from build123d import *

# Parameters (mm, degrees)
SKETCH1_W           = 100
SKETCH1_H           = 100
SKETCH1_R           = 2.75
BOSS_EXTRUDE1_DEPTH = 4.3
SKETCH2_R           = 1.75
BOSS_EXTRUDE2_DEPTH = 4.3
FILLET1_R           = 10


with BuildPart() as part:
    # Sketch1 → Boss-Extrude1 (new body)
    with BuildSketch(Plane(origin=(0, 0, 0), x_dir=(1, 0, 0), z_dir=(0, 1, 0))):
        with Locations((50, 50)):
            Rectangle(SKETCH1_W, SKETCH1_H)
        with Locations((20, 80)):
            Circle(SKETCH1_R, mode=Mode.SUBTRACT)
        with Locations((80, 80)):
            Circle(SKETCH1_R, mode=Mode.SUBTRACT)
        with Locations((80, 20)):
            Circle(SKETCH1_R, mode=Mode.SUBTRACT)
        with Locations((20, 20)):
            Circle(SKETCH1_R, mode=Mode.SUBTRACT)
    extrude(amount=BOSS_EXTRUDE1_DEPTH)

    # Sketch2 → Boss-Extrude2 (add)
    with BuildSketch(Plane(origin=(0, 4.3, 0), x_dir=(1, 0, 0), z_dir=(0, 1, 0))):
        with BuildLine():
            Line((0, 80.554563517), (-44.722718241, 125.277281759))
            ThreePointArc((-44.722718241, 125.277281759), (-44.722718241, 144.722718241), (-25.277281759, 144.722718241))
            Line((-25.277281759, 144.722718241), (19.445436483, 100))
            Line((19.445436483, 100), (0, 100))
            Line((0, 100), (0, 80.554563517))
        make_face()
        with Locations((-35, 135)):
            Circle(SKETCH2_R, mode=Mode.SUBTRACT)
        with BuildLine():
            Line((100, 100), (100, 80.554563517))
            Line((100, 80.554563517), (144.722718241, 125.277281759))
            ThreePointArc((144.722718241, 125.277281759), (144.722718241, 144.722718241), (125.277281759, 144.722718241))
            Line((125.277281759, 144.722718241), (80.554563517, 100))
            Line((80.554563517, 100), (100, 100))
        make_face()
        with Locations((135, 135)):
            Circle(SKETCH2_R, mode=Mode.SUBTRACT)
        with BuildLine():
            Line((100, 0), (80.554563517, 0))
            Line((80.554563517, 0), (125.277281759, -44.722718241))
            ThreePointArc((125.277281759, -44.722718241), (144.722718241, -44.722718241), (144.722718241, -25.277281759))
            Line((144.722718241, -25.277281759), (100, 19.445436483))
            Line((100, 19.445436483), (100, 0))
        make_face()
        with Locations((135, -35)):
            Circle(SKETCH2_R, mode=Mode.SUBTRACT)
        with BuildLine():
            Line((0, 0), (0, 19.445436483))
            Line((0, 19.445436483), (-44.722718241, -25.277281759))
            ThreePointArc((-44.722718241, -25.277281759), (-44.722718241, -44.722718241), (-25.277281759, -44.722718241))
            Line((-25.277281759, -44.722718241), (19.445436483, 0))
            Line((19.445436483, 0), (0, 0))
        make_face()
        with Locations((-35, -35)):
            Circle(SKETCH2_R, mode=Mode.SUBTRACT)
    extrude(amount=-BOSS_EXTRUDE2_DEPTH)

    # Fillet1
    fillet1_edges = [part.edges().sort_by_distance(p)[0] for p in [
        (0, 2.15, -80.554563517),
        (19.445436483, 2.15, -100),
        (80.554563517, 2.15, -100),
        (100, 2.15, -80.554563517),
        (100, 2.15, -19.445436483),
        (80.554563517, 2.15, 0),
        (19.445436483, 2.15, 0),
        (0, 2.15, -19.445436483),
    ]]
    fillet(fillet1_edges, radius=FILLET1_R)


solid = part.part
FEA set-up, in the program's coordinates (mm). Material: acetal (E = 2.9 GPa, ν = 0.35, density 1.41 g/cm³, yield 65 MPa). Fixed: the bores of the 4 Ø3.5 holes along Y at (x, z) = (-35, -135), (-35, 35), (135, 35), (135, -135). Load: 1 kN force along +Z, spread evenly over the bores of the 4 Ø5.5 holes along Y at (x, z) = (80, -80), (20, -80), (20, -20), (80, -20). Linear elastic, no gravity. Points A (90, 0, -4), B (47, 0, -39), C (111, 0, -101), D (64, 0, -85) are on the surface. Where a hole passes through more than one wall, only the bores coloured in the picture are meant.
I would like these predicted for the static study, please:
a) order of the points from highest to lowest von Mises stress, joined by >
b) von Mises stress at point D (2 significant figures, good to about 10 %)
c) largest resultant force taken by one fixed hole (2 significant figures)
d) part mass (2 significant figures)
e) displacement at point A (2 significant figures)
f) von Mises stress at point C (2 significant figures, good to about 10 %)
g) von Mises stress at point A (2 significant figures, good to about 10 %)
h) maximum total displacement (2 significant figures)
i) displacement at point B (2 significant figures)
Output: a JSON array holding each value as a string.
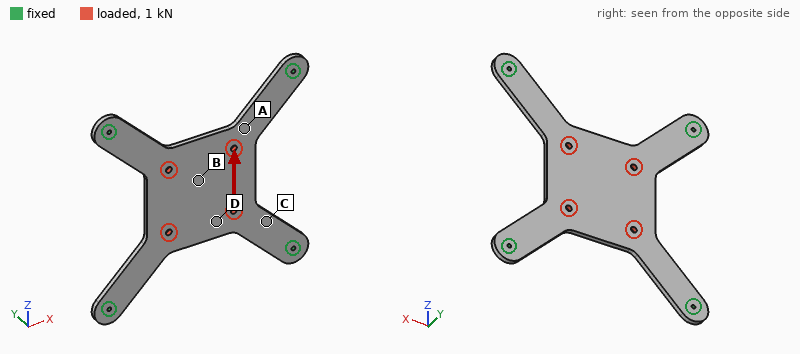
["C > A > D > B", "1.4 MPa", "340 N", "100 g", "0.12 mm", "3.3 MPa", "2.3 MPa", "0.14 mm", "0.12 mm"]
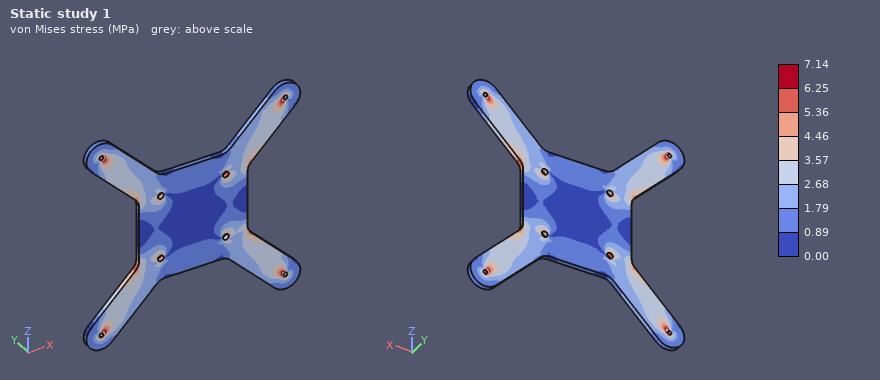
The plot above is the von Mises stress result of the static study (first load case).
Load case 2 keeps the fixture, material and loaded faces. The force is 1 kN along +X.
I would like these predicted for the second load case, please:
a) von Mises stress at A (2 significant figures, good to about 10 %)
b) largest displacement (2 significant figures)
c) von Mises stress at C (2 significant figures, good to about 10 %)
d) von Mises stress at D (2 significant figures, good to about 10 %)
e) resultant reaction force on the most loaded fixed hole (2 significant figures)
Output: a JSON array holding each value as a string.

["2.7 MPa", "0.14 mm", "2.4 MPa", "1.5 MPa", "340 N"]
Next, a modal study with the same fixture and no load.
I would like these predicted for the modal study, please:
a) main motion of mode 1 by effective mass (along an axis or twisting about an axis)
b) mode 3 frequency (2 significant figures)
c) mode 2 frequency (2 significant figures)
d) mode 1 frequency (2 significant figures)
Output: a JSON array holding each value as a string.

["along Y", "280 Hz", "280 Hz", "120 Hz"]
